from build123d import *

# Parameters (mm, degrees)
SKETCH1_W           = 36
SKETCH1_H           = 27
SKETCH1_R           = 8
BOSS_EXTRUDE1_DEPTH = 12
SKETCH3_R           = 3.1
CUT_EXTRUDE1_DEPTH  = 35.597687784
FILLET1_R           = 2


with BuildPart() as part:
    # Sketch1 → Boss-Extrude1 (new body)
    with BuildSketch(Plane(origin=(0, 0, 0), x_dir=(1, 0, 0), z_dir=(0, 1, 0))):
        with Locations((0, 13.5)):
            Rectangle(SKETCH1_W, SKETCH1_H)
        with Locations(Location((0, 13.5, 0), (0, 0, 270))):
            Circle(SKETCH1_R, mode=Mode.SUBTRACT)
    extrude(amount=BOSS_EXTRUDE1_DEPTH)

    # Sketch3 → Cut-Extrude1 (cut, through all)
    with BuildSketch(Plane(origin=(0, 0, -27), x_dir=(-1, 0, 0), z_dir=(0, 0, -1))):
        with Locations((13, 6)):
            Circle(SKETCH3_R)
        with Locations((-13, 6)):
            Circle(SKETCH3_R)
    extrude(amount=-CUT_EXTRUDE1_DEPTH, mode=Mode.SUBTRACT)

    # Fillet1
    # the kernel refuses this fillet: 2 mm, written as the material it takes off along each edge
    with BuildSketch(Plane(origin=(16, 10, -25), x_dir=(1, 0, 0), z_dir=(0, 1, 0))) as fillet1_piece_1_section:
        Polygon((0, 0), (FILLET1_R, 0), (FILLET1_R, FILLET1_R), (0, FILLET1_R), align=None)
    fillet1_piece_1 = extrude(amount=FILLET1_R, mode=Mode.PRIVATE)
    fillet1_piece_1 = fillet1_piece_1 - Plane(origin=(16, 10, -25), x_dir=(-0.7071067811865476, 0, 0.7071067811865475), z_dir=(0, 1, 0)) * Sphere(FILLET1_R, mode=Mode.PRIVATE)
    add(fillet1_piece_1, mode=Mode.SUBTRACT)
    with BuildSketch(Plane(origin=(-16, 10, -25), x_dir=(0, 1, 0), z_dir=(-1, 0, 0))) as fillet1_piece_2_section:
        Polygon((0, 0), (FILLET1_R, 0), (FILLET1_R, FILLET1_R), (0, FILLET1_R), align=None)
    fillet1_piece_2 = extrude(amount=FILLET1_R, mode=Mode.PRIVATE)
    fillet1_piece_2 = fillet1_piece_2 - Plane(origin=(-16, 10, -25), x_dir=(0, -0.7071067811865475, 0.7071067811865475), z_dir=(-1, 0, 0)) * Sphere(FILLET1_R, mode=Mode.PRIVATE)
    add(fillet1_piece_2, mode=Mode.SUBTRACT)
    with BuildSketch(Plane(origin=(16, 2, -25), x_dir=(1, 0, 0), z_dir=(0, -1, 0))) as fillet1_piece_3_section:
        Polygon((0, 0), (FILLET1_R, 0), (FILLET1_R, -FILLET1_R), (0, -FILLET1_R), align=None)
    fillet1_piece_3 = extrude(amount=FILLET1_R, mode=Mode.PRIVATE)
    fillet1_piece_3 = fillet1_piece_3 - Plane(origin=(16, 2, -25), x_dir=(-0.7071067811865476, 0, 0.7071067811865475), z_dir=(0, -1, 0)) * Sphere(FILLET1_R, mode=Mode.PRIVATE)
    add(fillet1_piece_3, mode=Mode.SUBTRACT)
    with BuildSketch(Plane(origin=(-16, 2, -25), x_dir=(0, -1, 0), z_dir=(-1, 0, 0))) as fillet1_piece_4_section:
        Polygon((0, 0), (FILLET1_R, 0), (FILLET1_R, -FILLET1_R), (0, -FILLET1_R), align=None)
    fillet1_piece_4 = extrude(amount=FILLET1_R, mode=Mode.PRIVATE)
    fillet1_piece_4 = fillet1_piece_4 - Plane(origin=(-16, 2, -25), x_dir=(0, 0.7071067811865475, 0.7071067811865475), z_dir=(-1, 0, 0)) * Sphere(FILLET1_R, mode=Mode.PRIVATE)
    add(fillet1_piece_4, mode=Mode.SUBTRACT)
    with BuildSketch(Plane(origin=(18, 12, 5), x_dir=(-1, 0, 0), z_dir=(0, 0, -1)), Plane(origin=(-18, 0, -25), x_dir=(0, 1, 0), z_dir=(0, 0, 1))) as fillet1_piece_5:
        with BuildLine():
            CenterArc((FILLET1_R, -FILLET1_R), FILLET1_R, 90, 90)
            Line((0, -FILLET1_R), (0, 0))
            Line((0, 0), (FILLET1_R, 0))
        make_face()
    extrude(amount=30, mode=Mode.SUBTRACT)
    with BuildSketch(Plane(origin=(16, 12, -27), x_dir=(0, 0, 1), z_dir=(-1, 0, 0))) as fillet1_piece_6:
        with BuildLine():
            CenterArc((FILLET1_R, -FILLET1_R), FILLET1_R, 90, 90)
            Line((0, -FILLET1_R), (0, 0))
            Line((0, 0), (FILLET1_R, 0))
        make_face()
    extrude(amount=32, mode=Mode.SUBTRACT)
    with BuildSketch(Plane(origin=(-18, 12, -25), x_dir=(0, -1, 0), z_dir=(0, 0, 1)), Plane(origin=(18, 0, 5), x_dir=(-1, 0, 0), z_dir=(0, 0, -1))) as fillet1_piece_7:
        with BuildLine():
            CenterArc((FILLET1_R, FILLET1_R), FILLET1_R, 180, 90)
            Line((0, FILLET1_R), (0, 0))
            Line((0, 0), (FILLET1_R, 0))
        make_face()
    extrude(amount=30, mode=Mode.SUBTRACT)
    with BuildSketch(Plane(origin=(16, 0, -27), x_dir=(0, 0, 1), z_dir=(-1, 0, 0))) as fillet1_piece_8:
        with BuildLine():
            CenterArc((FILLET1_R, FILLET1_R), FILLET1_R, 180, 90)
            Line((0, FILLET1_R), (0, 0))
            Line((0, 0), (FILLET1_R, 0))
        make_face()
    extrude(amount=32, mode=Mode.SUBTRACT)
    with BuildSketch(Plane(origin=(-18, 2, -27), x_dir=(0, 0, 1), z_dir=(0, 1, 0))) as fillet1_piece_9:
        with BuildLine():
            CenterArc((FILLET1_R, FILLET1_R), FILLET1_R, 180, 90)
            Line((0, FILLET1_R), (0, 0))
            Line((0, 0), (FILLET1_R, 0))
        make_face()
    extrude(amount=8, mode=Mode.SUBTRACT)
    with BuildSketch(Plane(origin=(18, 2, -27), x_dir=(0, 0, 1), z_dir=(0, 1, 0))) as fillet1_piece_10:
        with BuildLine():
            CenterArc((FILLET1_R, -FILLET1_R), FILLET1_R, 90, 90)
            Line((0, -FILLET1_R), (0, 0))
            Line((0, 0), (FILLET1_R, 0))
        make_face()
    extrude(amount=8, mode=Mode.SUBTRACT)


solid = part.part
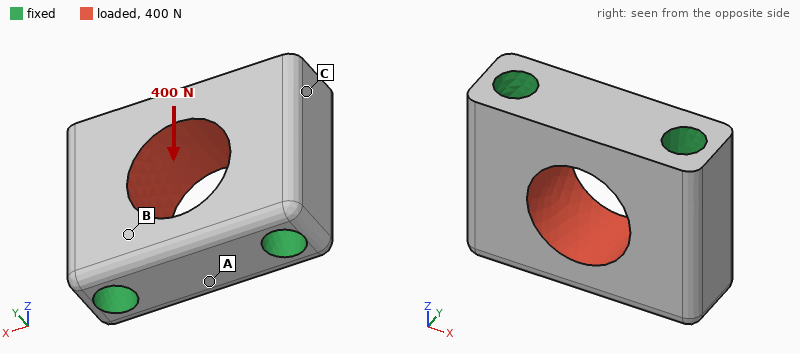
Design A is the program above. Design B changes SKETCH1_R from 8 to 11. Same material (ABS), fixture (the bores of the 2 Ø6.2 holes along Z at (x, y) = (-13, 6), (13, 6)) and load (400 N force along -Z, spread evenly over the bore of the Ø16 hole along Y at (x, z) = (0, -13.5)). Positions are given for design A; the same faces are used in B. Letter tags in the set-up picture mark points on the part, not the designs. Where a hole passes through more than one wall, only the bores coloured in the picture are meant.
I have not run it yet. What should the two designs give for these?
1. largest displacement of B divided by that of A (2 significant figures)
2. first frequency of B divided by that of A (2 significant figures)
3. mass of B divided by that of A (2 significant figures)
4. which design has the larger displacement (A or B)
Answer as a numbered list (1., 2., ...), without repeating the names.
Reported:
1. 2.5
2. 0.98
3. 0.72
4. B
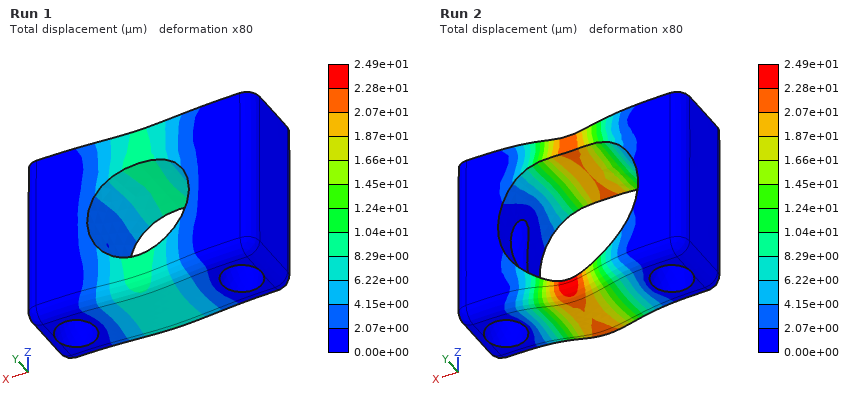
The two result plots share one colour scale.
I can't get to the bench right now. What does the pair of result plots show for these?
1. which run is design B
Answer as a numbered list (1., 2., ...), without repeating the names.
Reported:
1. Run 2
